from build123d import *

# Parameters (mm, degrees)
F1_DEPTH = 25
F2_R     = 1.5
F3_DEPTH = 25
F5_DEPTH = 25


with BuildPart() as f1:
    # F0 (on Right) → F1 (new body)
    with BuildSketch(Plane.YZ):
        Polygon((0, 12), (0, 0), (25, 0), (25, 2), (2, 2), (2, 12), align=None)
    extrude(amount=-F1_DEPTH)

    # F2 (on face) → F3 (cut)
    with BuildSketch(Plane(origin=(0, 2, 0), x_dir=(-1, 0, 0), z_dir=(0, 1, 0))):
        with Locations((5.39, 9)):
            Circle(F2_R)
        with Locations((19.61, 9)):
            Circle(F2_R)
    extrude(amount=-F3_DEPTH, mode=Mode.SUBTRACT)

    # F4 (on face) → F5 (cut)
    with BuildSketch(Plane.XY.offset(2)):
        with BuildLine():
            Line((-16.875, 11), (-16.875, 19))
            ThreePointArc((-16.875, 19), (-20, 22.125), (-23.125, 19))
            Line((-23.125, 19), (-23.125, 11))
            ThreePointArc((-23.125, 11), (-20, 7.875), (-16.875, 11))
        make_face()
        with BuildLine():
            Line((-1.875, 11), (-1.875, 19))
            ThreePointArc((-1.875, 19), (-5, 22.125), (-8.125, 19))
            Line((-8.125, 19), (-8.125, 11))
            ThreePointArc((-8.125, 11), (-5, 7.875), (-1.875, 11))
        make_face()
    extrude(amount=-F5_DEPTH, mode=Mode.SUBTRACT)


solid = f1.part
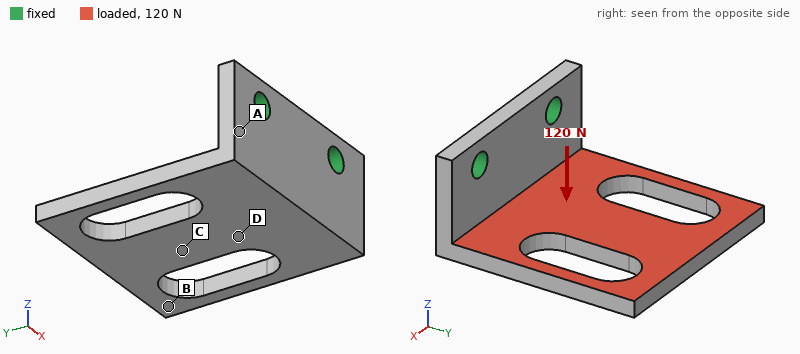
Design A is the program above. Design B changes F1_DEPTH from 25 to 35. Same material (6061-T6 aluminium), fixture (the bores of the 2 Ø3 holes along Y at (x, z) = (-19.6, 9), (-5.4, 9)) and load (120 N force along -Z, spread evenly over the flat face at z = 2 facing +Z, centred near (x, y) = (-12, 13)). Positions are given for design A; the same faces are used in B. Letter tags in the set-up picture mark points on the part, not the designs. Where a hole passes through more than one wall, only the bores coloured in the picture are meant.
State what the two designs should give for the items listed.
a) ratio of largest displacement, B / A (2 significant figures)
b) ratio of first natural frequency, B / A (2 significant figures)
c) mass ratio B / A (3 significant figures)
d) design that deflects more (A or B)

0.84
0.90
1.50
A
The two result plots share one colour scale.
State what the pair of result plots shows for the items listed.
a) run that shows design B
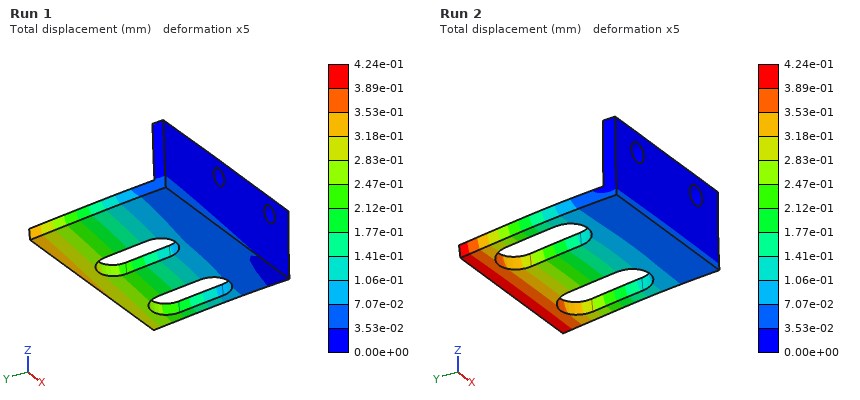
Run 1
